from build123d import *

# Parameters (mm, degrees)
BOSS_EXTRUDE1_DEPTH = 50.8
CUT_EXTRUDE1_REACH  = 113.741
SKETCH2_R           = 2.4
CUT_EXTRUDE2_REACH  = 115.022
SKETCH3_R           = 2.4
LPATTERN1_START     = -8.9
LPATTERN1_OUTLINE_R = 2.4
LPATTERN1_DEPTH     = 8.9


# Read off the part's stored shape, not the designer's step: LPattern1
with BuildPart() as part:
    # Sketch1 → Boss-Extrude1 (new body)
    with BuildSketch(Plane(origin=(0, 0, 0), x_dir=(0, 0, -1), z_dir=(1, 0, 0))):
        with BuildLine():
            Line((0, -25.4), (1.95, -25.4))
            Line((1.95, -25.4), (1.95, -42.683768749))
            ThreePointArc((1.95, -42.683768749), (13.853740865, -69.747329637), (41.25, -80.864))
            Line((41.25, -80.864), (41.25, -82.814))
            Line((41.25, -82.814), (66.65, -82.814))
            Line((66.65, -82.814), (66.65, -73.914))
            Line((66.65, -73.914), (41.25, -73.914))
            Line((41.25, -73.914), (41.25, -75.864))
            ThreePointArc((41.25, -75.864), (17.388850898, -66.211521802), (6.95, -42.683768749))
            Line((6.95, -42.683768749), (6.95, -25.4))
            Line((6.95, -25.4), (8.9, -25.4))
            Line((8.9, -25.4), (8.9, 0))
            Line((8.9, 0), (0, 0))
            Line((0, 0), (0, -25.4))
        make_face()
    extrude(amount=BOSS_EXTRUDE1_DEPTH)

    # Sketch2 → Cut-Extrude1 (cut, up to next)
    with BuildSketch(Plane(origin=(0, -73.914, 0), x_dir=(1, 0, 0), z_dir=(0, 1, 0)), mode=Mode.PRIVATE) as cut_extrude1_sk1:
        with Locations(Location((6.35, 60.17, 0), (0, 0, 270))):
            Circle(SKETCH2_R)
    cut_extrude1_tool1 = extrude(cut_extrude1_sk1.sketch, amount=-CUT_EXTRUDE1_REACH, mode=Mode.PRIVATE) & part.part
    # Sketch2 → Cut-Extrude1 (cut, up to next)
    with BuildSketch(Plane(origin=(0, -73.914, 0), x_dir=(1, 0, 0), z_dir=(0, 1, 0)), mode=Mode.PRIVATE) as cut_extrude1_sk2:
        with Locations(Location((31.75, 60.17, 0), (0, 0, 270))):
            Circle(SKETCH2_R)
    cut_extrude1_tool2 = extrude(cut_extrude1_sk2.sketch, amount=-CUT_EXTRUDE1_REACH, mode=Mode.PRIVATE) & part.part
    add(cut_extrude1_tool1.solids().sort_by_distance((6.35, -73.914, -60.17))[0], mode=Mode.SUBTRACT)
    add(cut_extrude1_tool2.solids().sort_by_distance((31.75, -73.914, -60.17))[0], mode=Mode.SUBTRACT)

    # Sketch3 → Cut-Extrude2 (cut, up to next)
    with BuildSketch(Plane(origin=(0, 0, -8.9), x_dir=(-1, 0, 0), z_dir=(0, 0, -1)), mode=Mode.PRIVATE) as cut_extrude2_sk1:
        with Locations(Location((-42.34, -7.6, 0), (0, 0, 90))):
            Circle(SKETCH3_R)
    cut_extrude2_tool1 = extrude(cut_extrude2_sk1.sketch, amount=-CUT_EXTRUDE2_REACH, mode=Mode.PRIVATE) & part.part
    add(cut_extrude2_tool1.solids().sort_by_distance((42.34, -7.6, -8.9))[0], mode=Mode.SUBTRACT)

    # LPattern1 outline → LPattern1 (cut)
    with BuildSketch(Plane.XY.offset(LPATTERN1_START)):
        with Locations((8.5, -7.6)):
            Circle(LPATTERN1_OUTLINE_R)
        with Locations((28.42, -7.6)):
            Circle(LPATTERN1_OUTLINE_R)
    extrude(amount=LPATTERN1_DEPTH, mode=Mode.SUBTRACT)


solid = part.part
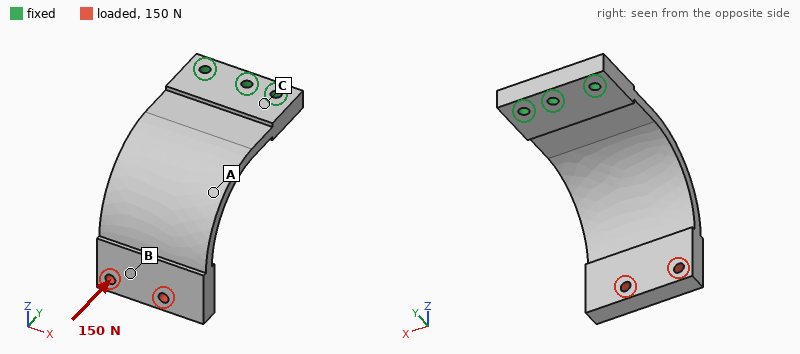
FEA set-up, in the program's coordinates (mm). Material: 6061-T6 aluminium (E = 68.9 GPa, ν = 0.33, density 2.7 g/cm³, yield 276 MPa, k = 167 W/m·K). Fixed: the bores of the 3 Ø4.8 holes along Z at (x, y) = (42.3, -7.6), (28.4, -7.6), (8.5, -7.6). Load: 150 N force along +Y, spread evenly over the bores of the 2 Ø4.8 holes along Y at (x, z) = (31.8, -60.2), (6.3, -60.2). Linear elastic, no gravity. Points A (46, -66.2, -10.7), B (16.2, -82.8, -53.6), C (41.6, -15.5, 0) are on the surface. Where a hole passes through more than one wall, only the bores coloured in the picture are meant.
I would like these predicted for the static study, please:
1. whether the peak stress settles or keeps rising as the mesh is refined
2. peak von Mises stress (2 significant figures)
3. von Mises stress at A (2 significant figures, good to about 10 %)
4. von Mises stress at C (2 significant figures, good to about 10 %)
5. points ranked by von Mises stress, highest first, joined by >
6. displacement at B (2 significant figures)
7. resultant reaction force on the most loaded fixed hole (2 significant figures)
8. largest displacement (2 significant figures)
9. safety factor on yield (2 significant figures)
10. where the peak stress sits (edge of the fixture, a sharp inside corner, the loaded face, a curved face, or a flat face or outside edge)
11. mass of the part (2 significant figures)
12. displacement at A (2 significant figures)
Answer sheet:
settles
43 MPa
31 MPa
13 MPa
A > C > B
0.72 mm
100 N
0.89 mm
6.4
a curved face
110 g
0.22 mm
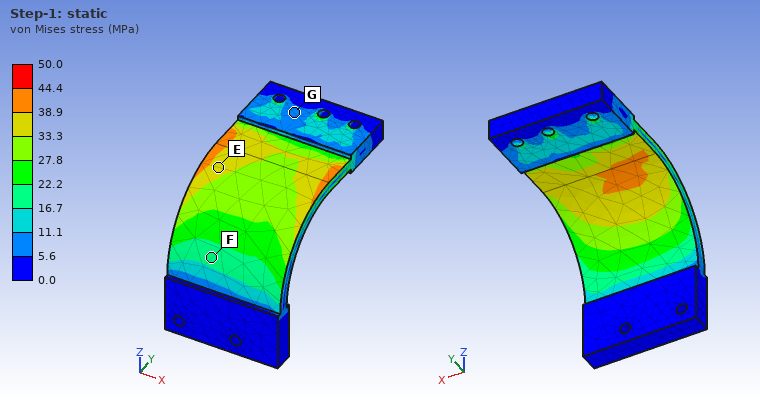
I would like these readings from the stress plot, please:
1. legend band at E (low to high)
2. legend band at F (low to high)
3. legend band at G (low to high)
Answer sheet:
33.3 to 38.9 MPa
16.7 to 22.2 MPa
5.6 to 11.1 MPa
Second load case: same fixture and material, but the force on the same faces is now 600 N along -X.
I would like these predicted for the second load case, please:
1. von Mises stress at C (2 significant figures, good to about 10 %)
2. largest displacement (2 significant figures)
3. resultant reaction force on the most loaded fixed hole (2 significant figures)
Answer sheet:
57 MPa
1.2 mm
1.5 kN
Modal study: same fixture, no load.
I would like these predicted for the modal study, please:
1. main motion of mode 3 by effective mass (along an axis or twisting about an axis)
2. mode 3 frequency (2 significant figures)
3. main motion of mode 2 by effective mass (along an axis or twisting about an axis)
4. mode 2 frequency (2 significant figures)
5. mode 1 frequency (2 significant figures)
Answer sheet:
along Z
1300 Hz
along X
700 Hz
360 Hz
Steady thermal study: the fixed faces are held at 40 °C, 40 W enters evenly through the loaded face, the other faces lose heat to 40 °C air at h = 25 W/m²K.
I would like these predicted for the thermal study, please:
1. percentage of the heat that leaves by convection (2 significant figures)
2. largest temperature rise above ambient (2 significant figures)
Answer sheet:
32 %
74 K
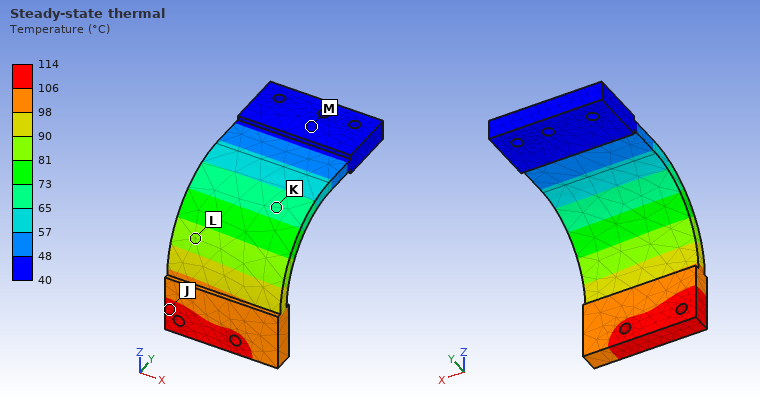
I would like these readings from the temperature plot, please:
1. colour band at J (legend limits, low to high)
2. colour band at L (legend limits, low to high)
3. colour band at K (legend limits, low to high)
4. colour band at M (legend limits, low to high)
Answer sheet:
106 to 114 °C
81 to 90 °C
65 to 73 °C
40 to 48 °C
